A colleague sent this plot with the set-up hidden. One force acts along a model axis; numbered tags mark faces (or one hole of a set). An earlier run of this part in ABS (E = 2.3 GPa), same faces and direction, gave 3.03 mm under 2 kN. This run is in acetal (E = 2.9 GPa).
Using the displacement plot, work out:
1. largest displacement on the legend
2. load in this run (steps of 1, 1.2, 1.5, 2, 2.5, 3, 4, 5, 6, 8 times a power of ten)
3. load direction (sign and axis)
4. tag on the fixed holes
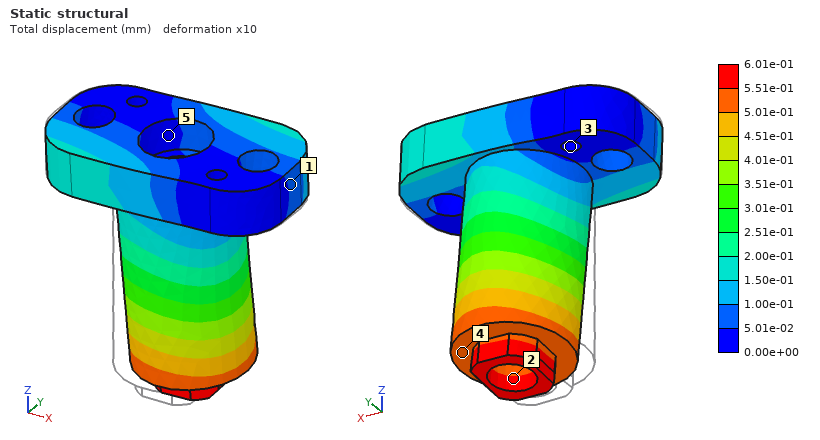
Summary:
6.01e-01 mm
500 N
+Y
3
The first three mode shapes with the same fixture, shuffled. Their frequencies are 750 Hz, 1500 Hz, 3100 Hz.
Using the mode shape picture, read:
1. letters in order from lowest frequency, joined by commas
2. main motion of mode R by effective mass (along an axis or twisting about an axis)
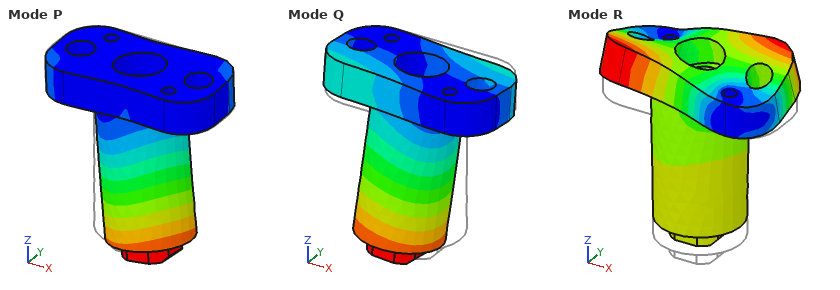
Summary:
Q, P, R
along Z
